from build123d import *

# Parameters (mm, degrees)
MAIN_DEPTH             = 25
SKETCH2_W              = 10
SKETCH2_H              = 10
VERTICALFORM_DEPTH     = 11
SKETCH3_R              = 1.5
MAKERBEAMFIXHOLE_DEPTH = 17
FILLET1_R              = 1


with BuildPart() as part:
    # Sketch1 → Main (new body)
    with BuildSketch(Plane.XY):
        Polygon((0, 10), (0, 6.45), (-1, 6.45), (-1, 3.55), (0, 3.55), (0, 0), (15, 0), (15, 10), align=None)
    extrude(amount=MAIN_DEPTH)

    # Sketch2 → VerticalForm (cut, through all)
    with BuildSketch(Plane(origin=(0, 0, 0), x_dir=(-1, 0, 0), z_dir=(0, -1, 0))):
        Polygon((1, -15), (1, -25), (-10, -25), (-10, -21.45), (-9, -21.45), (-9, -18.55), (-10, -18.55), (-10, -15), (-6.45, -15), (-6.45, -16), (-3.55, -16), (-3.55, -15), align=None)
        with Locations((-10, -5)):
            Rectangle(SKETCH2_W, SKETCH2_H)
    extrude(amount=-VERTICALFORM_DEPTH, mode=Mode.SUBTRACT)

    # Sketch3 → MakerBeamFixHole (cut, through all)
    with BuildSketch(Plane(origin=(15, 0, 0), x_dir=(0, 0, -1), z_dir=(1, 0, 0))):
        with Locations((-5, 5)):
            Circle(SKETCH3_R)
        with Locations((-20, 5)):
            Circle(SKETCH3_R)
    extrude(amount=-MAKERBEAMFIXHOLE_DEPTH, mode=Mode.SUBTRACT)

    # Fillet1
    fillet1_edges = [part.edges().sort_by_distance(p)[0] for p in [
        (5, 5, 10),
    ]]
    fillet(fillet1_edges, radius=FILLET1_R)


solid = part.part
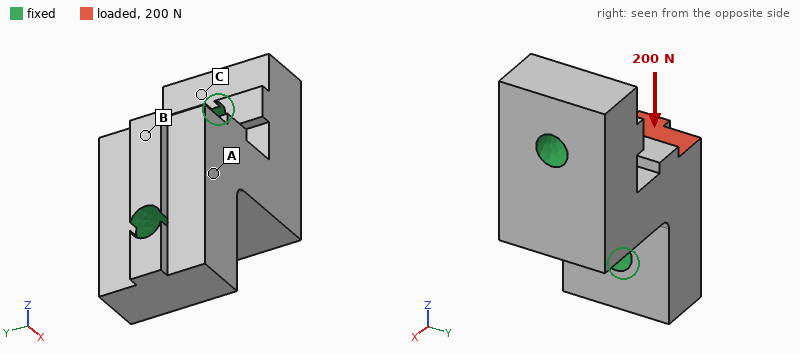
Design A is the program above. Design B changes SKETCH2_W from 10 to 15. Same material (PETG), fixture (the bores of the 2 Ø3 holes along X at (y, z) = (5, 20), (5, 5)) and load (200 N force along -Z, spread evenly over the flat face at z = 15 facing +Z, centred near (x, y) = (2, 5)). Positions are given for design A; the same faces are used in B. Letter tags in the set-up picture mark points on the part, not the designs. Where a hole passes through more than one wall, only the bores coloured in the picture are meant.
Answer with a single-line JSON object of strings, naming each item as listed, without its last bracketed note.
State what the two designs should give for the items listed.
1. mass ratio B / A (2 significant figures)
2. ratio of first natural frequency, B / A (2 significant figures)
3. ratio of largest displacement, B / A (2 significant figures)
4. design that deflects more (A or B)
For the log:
{"mass ratio B / A": "0.87", "ratio of first natural frequency, B / A": "0.87", "ratio of largest displacement, B / A": "1.2", "design that deflects more": "B"}
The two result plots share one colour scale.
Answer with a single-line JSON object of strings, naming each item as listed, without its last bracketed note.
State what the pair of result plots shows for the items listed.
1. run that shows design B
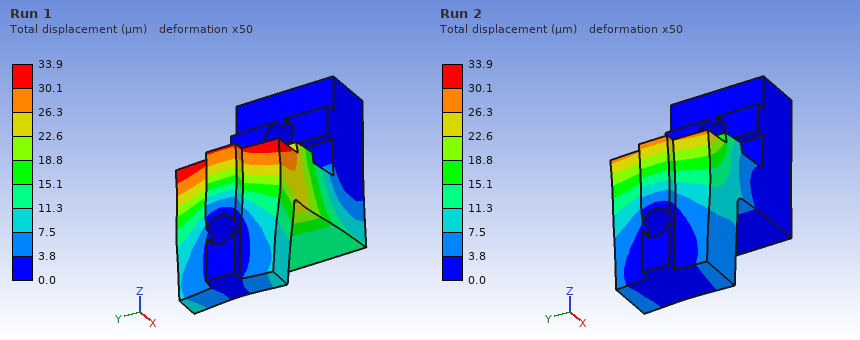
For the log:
{"run that shows design B": "Run 1"}
